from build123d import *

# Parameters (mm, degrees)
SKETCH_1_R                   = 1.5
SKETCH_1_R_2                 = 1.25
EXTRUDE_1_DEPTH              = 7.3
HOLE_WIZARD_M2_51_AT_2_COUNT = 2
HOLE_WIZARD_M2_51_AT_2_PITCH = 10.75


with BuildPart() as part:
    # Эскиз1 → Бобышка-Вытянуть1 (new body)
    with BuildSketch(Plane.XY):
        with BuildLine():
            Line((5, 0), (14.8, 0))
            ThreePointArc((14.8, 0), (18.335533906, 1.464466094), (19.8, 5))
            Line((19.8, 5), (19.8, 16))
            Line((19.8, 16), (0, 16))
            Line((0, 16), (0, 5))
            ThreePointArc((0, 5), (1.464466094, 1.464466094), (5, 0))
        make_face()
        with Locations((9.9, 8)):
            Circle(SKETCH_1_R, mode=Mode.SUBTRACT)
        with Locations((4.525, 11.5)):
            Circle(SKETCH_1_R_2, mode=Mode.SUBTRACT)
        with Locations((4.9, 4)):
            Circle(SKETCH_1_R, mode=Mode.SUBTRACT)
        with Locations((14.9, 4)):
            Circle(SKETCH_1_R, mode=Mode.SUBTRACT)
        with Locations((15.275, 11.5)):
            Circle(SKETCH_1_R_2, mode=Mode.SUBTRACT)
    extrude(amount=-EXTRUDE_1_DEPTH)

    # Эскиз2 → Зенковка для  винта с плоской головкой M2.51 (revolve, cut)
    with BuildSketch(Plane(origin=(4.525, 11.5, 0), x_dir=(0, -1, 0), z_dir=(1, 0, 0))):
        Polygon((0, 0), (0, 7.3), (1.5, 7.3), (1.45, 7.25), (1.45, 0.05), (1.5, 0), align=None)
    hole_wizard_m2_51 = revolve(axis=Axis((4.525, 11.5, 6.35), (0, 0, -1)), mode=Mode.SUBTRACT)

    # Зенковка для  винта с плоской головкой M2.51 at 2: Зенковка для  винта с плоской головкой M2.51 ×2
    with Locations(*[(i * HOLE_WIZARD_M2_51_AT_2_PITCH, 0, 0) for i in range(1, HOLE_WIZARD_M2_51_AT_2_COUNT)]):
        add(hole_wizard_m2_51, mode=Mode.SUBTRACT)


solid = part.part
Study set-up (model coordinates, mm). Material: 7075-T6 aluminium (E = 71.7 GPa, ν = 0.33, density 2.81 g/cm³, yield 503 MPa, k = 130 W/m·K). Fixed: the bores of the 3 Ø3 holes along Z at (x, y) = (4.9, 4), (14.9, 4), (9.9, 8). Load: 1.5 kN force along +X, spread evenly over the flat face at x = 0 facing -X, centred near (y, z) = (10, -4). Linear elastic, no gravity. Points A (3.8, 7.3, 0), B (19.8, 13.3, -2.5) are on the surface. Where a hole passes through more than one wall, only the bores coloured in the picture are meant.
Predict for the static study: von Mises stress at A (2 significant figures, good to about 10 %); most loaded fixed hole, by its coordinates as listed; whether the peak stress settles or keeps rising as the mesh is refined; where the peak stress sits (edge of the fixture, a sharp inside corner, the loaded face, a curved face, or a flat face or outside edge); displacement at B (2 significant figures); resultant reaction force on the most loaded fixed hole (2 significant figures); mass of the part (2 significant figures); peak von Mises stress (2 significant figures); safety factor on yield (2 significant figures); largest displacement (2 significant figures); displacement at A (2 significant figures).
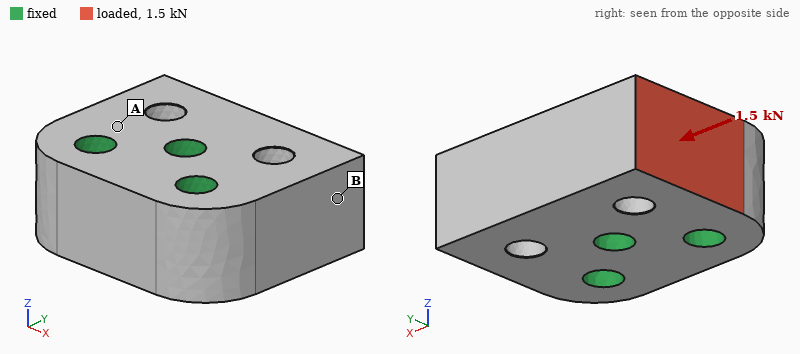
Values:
20 MPa
(9.9, 8)
settles
a curved face
2.3 µm
1.1 kN
5.6 g
70 MPa
7.2
6.2 µm
1.3 µm
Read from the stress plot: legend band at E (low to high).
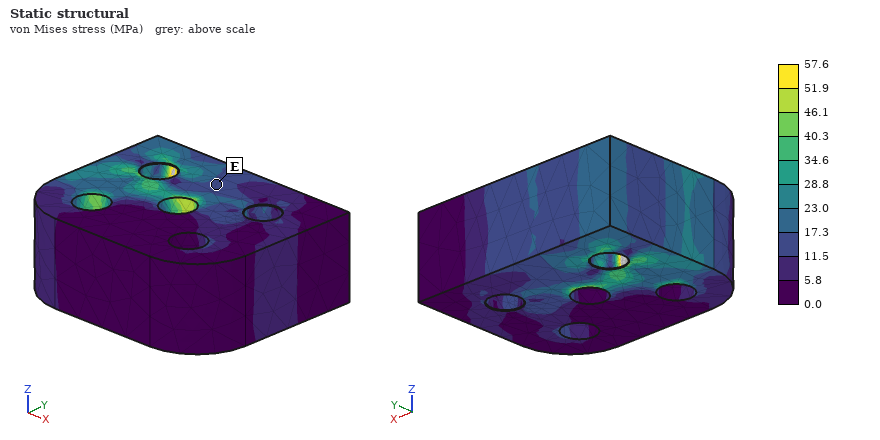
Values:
11.5 to 17.3 MPa
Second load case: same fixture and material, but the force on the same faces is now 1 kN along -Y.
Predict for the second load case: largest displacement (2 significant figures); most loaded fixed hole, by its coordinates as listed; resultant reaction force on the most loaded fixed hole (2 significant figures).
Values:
7.0 µm
(4.9, 4)
1.2 kN
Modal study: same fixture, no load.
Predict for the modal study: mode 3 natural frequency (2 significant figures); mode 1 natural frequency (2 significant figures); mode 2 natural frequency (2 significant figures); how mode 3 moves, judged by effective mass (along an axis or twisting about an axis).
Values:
58 kHz
50 kHz
52 kHz
along X
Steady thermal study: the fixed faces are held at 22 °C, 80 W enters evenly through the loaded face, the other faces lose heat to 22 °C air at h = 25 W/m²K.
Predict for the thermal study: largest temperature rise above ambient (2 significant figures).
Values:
69 K
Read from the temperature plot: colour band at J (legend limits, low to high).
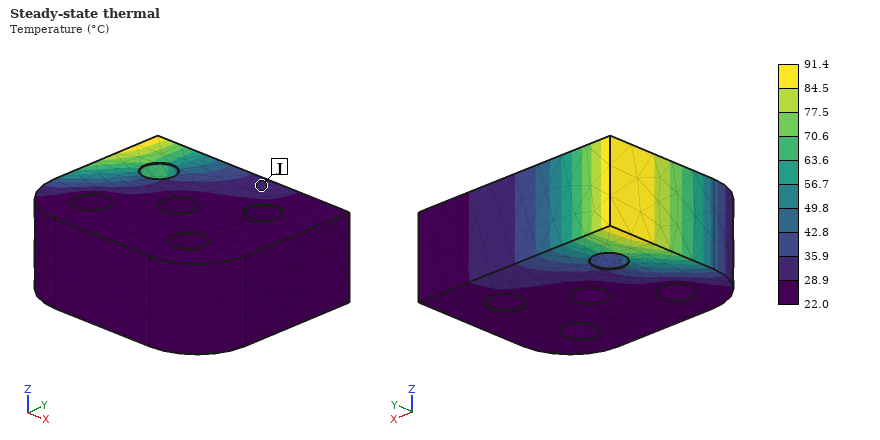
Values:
28.9 to 35.9 °C
